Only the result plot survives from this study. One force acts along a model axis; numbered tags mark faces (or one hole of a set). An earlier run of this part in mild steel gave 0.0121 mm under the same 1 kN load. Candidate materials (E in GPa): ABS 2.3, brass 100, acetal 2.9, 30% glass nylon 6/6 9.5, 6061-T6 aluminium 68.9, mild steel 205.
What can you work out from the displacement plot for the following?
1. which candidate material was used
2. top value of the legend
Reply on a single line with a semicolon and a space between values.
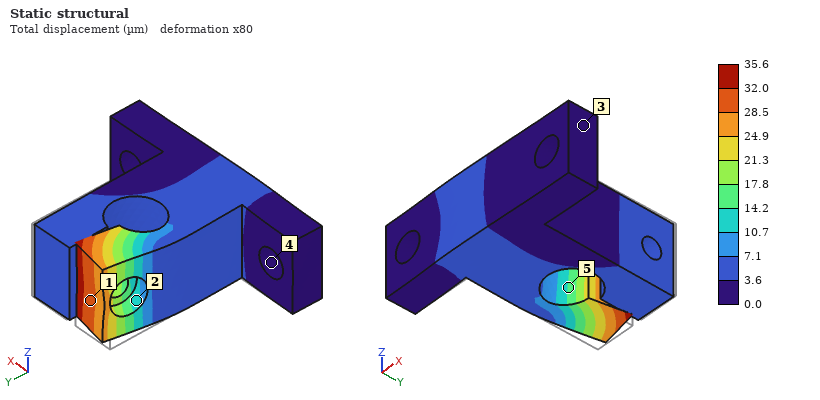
6061-T6 aluminium; 35.6 µm
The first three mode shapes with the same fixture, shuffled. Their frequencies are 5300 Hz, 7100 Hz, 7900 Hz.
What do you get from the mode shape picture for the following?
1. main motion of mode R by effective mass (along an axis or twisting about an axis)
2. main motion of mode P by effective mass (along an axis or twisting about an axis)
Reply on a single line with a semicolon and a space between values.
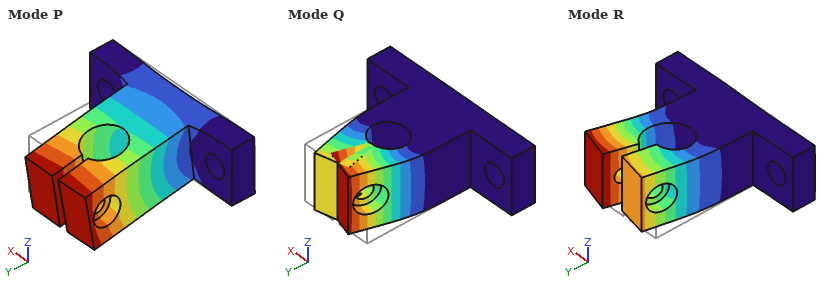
along X; along Z
